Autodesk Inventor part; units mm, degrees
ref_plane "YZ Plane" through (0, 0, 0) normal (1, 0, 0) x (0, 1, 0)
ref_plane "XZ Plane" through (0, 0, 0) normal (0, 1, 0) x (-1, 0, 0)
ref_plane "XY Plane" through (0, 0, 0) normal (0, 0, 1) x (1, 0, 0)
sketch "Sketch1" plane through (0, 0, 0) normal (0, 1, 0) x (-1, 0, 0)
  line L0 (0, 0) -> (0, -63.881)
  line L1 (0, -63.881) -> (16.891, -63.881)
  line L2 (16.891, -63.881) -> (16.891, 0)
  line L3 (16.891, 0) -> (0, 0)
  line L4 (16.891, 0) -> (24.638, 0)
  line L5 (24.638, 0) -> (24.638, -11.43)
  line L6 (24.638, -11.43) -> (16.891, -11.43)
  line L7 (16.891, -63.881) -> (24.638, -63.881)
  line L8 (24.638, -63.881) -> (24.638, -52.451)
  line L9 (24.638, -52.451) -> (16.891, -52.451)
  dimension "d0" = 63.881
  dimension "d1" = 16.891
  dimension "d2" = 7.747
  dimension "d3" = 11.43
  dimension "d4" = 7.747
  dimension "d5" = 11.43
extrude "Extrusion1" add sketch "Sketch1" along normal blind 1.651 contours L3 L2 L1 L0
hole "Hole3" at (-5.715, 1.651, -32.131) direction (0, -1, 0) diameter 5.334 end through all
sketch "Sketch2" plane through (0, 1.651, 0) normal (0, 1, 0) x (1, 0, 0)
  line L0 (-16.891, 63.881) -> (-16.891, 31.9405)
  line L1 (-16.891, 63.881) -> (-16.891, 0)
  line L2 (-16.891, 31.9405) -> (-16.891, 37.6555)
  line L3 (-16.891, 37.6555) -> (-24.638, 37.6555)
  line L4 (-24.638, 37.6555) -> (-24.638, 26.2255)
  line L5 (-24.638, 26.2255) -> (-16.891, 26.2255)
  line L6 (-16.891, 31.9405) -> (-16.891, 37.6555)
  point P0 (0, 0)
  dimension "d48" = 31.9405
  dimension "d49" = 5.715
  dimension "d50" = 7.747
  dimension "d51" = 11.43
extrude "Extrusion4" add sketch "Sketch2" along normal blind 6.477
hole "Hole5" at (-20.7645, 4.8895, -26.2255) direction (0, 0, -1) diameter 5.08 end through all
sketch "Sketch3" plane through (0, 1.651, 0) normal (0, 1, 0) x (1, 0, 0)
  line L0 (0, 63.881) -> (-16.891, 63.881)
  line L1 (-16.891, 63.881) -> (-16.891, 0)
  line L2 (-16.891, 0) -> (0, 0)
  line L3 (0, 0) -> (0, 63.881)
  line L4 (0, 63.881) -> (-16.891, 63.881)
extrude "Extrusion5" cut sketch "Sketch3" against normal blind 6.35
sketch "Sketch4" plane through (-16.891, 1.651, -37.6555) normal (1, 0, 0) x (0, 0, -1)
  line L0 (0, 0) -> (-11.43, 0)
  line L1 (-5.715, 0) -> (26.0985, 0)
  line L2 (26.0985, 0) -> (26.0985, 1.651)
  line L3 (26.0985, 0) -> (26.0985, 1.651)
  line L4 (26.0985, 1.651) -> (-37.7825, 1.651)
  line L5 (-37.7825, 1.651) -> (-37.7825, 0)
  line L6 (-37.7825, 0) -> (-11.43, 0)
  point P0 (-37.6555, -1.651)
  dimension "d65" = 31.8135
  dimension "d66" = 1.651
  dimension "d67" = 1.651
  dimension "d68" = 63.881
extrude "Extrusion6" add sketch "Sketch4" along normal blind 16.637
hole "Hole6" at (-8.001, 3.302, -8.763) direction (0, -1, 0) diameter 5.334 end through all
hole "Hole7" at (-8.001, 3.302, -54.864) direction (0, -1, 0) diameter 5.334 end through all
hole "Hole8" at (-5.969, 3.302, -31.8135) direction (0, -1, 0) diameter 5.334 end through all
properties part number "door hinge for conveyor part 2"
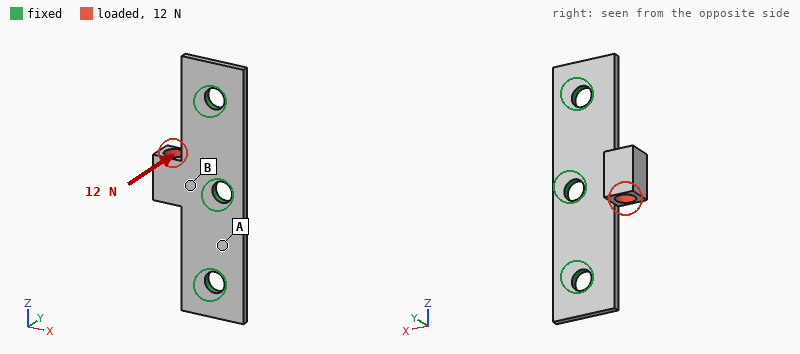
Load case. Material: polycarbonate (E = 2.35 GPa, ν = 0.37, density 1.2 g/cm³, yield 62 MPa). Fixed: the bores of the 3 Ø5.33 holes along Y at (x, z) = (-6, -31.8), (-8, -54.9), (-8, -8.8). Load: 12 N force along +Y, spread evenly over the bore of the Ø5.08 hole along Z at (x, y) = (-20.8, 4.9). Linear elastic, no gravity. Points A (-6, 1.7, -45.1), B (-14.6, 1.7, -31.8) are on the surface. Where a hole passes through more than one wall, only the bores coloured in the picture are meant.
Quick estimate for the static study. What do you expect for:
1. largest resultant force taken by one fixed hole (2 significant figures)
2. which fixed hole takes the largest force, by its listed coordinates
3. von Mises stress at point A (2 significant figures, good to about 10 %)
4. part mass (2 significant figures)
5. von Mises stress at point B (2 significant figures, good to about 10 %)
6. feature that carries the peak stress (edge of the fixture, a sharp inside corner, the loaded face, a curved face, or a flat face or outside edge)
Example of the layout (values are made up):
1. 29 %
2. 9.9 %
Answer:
1. 11 N
2. (-6, -31.8)
3. 1.8 MPa
4. 2.4 g
5. 7.9 MPa
6. a flat face or outside edge
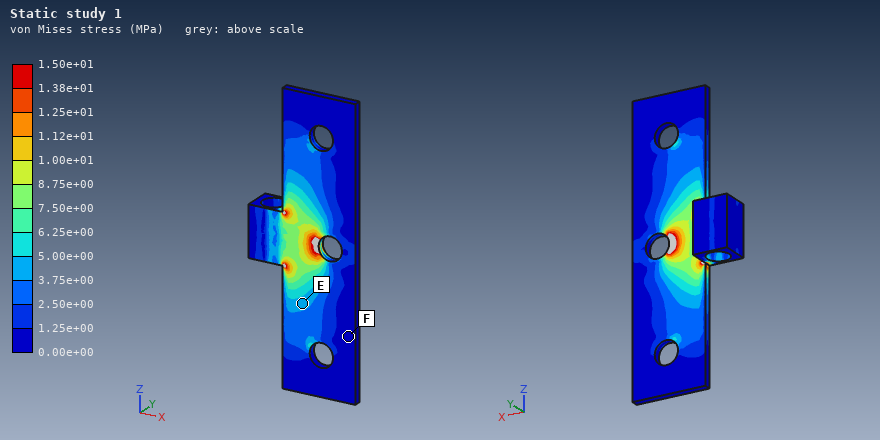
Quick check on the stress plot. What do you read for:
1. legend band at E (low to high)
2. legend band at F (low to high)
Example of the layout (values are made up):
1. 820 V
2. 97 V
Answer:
1. 3.75e+00 to 5.00e+00 MPa
2. 0.00e+00 to 1.25e+00 MPa
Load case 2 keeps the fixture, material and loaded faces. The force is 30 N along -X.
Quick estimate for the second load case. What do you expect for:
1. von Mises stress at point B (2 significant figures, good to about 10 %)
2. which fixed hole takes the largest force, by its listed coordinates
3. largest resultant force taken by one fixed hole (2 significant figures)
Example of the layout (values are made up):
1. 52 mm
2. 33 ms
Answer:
1. 7.5 MPa
2. (-6, -31.8)
3. 26 N
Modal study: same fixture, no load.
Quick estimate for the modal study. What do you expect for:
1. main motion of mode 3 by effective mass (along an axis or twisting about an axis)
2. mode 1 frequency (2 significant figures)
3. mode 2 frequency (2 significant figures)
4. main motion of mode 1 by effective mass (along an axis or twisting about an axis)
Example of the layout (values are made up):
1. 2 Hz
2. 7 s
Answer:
1. along Y
2. 1100 Hz
3. 3100 Hz
4. along Y
